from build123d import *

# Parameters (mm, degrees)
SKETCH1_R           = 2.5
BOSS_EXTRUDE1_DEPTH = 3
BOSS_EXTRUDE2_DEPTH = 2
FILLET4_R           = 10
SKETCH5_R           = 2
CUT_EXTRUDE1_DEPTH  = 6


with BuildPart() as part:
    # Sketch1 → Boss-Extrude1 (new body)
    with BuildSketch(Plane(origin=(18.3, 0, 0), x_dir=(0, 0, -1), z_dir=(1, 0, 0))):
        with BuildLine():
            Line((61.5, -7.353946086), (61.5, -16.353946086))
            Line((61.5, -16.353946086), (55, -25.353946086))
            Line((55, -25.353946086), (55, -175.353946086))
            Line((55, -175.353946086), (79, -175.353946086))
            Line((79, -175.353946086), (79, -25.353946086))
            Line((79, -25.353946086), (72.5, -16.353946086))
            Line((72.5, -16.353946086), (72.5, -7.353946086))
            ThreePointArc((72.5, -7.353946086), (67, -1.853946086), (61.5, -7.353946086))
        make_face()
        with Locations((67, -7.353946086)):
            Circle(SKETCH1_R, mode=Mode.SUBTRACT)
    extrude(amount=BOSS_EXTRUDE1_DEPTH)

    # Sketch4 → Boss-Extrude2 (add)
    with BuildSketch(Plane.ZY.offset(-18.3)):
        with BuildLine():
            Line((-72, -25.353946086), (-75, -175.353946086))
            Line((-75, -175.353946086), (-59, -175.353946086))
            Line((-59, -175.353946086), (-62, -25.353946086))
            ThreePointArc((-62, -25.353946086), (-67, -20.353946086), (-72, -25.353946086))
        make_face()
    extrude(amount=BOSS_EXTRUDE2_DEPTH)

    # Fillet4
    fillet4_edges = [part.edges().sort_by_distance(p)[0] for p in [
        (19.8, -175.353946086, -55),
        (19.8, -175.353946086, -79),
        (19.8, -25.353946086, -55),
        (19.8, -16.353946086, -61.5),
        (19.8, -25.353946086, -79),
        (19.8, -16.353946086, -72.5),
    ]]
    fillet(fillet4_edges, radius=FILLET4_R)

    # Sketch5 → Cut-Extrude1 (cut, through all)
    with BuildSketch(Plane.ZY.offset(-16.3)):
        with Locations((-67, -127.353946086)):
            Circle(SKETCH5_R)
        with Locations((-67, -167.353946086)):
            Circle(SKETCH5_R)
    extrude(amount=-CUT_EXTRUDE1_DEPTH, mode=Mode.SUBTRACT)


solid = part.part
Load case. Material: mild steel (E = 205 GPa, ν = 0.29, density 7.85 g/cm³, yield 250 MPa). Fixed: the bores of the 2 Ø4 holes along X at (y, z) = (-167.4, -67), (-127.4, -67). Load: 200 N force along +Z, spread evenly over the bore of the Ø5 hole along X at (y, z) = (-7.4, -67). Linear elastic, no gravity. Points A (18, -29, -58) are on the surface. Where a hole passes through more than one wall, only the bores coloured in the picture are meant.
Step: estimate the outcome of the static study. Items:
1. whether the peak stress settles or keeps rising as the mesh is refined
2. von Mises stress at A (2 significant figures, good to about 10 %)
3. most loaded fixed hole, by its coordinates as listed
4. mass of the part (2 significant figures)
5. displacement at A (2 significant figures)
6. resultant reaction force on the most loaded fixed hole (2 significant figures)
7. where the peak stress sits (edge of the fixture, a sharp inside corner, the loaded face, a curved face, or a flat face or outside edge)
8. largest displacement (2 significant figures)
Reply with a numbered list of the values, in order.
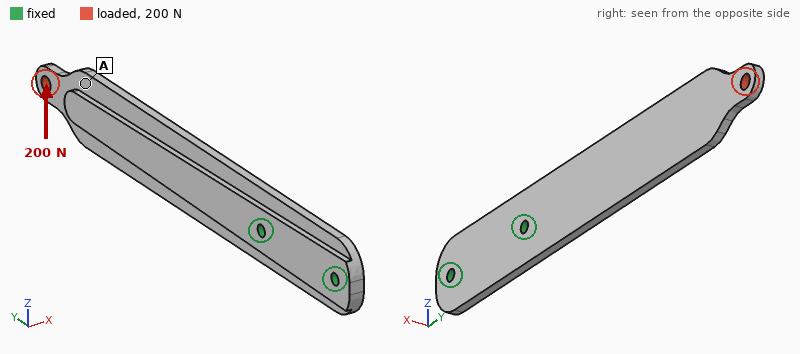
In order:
1. keeps rising
2. 11 MPa
3. (-127.4, -67)
4. 120 g
5. 0.14 mm
6. 660 N
7. edge of the fixture
8. 0.21 mm
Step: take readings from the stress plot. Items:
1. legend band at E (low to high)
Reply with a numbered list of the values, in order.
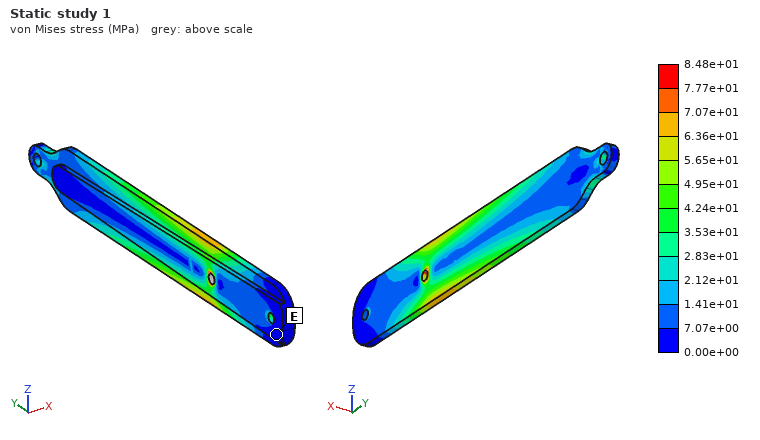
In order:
1. 0.00e+00 to 7.07e+00 MPa
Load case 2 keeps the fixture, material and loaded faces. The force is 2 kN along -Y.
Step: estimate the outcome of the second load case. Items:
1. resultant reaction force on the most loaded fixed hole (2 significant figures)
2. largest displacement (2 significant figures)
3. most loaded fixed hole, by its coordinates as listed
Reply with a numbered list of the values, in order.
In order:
1. 1.8 kN
2. 0.28 mm
3. (-127.4, -67)
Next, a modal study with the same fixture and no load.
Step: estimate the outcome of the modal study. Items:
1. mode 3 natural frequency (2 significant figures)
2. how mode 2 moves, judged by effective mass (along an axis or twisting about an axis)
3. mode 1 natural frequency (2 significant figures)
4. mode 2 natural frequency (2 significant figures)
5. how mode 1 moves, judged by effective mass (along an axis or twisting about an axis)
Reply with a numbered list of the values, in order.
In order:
1. 1800 Hz
2. along Z
3. 310 Hz
4. 1200 Hz
5. along X
